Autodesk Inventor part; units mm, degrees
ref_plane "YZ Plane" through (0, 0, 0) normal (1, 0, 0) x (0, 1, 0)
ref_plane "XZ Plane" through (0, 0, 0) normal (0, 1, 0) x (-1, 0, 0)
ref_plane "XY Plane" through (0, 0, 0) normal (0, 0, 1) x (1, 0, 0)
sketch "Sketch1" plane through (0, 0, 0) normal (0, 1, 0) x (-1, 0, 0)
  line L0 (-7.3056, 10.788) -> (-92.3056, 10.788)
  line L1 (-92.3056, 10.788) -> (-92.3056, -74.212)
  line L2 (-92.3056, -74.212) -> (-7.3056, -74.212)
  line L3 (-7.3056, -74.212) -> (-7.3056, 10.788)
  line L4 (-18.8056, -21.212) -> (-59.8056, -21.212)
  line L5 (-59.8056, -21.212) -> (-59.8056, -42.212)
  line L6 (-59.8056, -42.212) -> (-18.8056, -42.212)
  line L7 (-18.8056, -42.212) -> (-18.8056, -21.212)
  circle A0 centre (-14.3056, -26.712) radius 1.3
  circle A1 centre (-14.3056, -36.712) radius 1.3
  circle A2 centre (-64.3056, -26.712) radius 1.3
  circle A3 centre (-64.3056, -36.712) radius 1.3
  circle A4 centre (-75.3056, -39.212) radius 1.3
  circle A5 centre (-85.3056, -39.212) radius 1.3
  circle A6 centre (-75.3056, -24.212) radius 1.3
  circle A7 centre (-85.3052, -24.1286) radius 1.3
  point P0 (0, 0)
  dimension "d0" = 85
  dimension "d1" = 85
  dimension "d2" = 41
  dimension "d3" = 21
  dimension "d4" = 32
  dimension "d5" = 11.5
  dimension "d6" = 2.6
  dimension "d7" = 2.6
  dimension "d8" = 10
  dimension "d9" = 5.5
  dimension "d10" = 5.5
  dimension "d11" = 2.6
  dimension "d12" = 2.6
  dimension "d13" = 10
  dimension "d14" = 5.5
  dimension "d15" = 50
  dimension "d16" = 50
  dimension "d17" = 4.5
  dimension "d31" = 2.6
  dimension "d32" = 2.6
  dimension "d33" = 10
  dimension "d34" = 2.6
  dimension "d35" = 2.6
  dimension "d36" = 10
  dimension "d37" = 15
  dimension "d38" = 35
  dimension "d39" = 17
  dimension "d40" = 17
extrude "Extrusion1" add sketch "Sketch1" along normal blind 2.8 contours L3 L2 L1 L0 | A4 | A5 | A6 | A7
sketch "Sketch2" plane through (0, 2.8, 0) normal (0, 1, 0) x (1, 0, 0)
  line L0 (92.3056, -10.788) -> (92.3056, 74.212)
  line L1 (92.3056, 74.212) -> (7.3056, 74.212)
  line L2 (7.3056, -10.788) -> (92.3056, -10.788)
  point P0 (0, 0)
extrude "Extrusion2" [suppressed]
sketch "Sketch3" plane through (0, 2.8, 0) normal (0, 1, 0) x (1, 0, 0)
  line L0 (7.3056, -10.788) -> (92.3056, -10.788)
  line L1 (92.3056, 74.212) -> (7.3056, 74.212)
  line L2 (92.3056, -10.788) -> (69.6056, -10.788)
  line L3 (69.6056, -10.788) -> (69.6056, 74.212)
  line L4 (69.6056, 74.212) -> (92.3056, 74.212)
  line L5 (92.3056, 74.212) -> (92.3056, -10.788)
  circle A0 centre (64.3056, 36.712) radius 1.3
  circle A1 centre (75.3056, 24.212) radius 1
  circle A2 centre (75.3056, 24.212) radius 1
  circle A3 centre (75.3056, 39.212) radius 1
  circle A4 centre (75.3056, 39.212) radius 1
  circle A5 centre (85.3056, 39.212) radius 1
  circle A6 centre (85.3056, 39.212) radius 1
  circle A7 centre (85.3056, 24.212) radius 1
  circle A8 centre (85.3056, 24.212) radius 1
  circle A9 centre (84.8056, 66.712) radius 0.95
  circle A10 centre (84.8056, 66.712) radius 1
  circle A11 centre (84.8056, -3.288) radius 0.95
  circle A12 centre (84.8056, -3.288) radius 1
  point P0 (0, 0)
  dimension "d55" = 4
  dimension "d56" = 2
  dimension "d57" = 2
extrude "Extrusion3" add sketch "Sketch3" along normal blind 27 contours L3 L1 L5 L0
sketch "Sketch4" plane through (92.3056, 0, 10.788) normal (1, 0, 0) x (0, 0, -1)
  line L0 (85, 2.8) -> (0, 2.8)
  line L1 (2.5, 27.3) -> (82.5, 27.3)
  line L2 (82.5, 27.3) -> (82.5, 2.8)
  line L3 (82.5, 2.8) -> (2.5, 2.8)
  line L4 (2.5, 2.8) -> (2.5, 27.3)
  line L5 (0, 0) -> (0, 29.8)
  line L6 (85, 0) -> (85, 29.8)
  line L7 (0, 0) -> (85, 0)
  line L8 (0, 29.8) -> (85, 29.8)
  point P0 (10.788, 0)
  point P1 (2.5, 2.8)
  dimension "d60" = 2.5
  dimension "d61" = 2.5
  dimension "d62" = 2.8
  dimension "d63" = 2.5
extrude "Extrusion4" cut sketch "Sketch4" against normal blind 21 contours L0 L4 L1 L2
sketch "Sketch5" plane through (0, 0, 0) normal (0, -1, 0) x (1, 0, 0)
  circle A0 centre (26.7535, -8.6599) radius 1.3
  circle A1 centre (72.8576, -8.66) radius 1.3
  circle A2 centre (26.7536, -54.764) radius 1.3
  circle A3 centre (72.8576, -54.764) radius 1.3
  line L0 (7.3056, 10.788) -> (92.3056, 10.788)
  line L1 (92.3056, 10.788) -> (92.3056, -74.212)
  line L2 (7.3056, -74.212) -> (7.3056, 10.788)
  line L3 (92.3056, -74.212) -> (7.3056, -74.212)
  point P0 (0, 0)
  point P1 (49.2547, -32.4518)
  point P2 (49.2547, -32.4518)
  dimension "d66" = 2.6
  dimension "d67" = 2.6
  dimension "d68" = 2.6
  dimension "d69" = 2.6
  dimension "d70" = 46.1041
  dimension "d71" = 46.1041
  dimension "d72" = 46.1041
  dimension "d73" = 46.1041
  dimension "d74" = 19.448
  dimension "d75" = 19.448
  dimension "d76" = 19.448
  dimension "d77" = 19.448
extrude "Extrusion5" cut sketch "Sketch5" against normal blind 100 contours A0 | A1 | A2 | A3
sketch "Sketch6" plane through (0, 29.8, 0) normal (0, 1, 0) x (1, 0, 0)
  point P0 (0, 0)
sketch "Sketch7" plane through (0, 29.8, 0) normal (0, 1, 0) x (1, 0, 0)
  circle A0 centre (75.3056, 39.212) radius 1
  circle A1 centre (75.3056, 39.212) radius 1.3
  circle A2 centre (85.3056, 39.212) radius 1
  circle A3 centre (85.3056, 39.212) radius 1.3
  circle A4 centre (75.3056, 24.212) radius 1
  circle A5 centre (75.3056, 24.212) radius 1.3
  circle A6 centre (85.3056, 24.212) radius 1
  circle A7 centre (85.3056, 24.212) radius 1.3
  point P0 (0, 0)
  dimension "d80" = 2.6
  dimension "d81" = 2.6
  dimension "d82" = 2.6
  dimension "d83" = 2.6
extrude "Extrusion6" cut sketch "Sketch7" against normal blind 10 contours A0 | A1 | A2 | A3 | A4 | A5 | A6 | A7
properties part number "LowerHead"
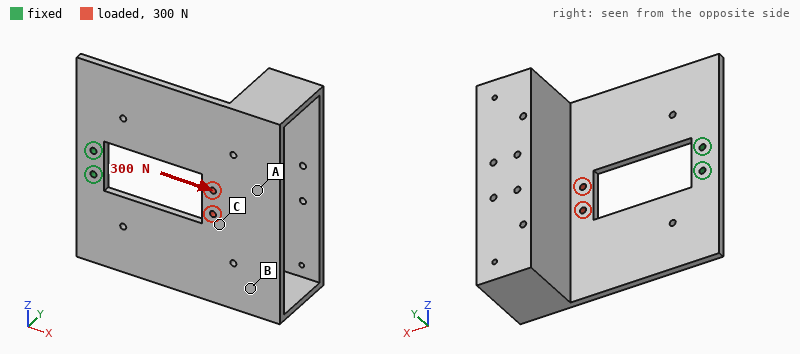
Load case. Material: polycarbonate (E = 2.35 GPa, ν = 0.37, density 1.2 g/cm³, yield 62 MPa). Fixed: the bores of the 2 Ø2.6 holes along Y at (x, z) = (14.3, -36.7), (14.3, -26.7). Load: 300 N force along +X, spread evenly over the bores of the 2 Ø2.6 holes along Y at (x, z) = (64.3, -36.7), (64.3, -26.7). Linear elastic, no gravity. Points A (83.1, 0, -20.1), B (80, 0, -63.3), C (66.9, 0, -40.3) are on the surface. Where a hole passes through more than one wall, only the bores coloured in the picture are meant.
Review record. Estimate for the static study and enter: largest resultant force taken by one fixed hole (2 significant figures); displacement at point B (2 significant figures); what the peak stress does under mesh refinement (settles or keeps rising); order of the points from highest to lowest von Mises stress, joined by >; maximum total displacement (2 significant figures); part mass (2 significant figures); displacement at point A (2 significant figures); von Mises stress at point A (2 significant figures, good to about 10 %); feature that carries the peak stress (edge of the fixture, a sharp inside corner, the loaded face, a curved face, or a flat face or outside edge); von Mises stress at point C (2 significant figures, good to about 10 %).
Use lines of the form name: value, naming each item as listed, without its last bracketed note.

largest resultant force taken by one fixed hole: 150 N
displacement at point B: 0.16 mm
what the peak stress does under mesh refinement: keeps rising
order of the points from highest to lowest von Mises stress, joined by >: C > A > B
maximum total displacement: 0.24 mm
part mass: 34 g
displacement at point A: 0.21 mm
von Mises stress at point A: 2.2 MPa
feature that carries the peak stress: edge of the fixture
von Mises stress at point C: 5.2 MPa
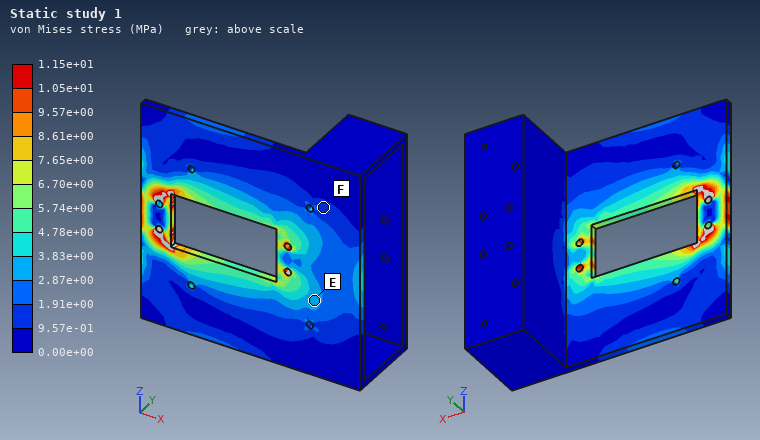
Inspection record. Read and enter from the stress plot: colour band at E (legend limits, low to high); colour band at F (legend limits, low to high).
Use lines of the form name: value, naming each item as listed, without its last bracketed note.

colour band at E: 2.87e+00 to 3.83e+00 MPa
colour band at F: 9.57e-01 to 1.91e+00 MPa
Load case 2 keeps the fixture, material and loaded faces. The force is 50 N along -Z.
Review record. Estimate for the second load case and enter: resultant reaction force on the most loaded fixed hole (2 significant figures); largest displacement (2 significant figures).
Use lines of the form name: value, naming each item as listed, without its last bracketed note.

resultant reaction force on the most loaded fixed hole: 180 N
largest displacement: 1.3 mm
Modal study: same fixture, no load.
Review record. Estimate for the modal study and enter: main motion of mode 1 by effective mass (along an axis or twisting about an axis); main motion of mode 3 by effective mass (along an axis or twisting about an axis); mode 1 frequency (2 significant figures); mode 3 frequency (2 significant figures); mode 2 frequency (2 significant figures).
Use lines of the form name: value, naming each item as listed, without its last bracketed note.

main motion of mode 1 by effective mass: along Y
main motion of mode 3 by effective mass: along Z
mode 1 frequency: 38 Hz
mode 3 frequency: 200 Hz
mode 2 frequency: 75 Hz
